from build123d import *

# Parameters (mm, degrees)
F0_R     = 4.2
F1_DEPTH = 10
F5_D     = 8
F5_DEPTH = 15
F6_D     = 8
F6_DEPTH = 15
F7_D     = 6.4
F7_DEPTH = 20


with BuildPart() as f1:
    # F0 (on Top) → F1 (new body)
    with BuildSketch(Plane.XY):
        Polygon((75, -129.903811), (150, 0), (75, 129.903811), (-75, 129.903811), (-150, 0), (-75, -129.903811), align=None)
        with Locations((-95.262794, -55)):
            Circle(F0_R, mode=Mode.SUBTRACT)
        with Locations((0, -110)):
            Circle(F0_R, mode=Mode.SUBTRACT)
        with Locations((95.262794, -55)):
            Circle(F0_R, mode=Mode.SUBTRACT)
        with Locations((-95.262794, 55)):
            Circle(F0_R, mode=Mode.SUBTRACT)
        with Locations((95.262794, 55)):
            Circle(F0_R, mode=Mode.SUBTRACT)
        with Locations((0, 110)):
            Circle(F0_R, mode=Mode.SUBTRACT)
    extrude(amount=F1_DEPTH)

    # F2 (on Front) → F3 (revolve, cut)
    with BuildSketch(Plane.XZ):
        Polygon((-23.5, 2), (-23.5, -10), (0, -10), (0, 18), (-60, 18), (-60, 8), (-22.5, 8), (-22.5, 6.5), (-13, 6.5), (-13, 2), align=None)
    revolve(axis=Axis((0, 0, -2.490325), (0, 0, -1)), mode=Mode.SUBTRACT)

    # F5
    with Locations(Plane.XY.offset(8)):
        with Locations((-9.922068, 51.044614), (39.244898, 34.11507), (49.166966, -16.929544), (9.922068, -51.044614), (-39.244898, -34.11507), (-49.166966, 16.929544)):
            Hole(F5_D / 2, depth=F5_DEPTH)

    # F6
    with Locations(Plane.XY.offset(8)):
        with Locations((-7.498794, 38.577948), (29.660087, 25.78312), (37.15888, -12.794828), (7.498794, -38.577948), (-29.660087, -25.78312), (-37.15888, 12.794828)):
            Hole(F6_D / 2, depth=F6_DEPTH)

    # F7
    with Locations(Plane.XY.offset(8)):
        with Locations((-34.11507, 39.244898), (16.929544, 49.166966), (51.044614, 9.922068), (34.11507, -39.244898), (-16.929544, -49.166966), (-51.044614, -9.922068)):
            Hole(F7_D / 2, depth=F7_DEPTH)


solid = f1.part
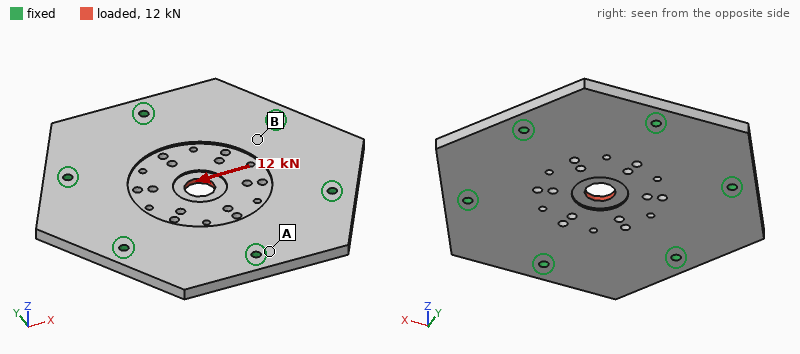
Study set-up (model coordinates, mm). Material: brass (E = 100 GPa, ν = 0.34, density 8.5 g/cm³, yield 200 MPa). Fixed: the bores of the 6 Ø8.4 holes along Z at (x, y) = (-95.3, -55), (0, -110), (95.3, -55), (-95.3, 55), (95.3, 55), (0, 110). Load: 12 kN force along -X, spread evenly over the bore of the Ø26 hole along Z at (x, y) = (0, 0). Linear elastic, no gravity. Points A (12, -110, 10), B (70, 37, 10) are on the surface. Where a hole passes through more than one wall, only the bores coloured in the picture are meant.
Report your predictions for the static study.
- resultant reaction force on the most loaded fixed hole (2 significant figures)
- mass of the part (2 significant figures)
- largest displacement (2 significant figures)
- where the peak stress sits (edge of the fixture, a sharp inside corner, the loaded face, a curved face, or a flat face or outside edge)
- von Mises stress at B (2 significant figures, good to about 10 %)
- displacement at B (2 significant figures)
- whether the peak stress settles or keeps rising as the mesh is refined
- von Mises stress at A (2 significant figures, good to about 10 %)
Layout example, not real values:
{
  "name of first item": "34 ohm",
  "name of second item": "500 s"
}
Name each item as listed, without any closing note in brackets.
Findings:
{
  "resultant reaction force on the most loaded fixed hole": "2.6 kN",
  "mass of the part": "4.6 kg",
  "largest displacement": "12 µm",
  "where the peak stress sits": "a sharp inside corner",
  "von Mises stress at B": "5.3 MPa",
  "displacement at B": "2.3 µm",
  "whether the peak stress settles or keeps rising as the mesh is refined": "keeps rising",
  "von Mises stress at A": "2.5 MPa"
}
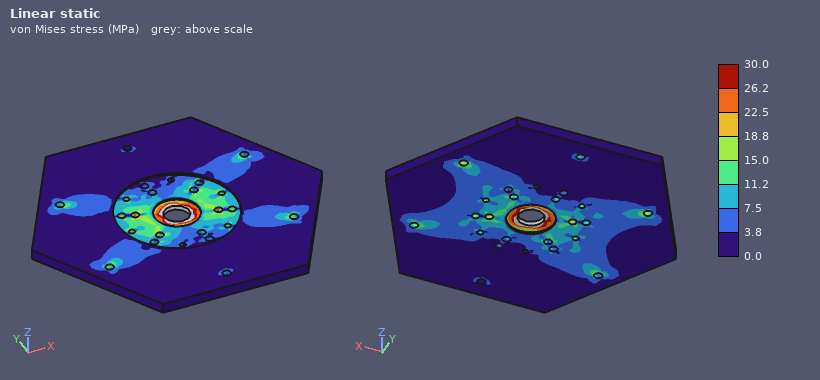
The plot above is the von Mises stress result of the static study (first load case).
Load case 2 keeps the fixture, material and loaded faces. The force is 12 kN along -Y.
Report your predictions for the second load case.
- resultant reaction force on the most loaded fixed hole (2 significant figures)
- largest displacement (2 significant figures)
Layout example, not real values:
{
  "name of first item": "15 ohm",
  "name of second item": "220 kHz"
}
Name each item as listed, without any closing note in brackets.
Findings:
{
  "resultant reaction force on the most loaded fixed hole": "3.0 kN",
  "largest displacement": "12 µm"
}
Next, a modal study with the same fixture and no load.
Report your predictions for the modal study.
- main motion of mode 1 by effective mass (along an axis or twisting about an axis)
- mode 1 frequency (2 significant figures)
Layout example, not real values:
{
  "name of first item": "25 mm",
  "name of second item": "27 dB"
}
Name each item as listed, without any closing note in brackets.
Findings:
{
  "main motion of mode 1 by effective mass": "along Z",
  "mode 1 frequency": "1100 Hz"
}
